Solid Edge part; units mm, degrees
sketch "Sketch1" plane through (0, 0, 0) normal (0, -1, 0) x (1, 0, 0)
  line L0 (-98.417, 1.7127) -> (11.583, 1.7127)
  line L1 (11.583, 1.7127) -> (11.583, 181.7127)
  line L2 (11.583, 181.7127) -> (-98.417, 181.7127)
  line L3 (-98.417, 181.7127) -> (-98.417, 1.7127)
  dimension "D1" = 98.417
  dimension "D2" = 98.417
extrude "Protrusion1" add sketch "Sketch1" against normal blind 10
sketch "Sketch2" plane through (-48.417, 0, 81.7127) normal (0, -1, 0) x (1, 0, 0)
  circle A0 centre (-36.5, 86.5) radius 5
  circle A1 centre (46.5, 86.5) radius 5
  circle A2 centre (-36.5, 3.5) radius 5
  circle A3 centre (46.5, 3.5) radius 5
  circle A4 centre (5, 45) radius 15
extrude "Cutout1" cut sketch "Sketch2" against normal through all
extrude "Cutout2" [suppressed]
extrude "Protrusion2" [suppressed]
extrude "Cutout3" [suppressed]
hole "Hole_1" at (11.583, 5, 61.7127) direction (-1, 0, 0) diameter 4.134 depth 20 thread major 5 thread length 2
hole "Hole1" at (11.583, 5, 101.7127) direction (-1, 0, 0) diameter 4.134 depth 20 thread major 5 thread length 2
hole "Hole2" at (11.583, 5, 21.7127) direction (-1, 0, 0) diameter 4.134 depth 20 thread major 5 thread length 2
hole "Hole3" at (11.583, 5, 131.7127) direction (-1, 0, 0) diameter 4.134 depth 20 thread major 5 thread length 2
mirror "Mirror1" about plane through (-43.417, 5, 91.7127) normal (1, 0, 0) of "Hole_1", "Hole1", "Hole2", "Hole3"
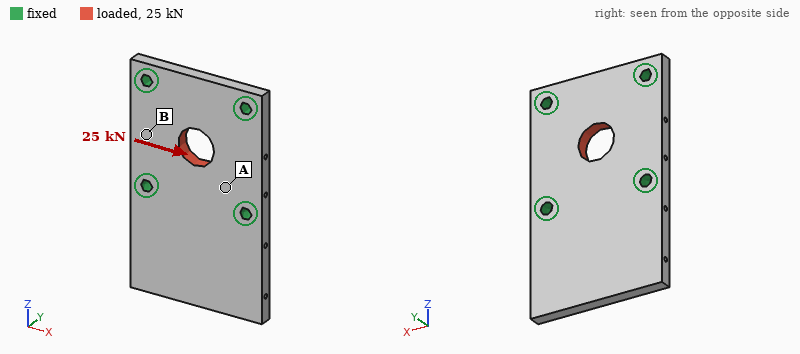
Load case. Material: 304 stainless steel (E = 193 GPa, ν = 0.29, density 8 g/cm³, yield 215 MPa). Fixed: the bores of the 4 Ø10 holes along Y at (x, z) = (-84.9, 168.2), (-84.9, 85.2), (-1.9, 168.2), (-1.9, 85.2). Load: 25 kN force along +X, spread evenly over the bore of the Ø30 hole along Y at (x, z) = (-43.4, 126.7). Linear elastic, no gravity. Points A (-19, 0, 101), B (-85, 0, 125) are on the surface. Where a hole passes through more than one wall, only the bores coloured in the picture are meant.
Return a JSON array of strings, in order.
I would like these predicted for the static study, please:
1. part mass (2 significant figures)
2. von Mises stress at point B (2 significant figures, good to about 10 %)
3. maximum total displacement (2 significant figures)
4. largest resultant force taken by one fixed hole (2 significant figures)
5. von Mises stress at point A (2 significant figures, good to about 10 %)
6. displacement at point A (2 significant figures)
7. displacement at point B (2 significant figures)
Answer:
["1.5 kg", "8.0 MPa", "7.9 µm", "6.9 kN", "26 MPa", "3.4 µm", "5.8 µm"]
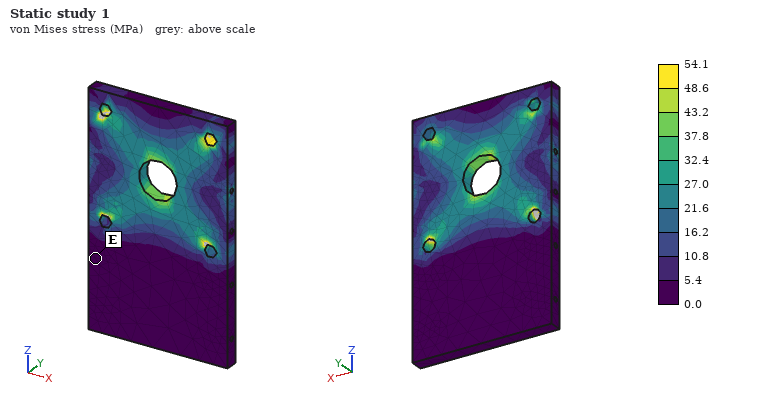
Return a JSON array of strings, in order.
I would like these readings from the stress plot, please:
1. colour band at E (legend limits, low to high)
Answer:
["0.0 to 5.4 MPa"]
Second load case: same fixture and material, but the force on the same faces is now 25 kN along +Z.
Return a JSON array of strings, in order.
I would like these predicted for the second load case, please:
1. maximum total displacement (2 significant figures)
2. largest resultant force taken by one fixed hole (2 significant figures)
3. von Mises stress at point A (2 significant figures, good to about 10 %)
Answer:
["7.7 µm", "7.0 kN", "21 MPa"]
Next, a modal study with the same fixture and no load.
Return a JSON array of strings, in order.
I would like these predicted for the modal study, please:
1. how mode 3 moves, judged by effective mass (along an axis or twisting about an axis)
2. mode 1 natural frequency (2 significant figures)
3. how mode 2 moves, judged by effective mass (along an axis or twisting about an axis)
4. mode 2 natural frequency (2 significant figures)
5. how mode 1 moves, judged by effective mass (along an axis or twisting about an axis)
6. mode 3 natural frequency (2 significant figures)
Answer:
["along Y", "1100 Hz", "twisting about Z", "2300 Hz", "along Y", "5200 Hz"]
